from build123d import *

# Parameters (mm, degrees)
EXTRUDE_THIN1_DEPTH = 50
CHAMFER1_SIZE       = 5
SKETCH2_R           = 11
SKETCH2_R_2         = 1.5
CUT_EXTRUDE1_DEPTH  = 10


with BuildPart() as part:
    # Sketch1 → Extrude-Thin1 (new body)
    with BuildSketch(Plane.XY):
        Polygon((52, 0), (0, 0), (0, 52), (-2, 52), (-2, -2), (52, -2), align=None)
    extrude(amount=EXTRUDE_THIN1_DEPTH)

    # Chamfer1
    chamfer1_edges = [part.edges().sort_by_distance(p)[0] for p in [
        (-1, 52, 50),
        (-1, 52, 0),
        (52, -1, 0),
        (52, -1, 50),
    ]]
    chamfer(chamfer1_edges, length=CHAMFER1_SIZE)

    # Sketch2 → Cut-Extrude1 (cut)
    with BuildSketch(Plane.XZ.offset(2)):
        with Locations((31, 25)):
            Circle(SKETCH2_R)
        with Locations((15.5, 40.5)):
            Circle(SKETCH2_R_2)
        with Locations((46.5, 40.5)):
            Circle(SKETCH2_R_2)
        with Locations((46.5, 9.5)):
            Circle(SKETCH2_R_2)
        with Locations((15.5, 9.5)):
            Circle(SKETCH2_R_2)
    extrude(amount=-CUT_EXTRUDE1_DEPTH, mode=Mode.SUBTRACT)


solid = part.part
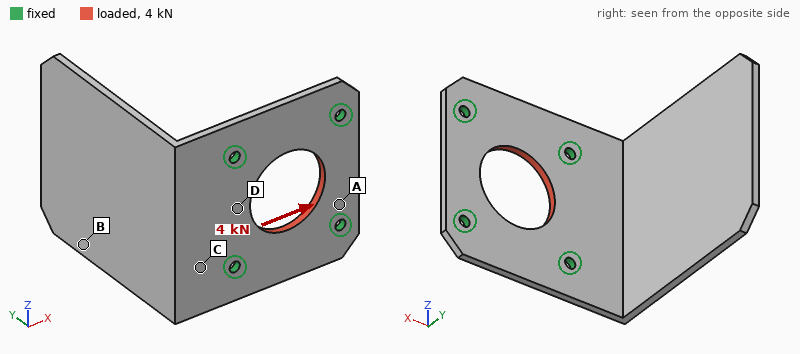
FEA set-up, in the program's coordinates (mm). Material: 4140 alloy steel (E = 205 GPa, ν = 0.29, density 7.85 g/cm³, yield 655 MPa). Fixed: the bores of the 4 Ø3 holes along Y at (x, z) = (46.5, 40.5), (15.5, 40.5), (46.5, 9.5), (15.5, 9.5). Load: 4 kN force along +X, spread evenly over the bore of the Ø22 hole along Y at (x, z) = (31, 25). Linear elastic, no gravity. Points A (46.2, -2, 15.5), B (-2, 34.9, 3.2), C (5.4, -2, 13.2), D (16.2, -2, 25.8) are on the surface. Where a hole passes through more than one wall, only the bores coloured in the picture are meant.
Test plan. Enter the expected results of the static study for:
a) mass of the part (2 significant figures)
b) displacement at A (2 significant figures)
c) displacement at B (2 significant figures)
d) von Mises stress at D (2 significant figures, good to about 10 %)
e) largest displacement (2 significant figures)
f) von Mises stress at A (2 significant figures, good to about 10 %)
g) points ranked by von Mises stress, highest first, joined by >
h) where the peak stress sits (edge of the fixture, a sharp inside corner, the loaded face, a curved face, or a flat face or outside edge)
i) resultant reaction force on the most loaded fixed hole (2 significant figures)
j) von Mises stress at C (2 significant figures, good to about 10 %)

76 g
2.8 µm
1.6 µm
24 MPa
6.3 µm
41 MPa
A > D > C > B
edge of the fixture
1.0 kN
14 MPa
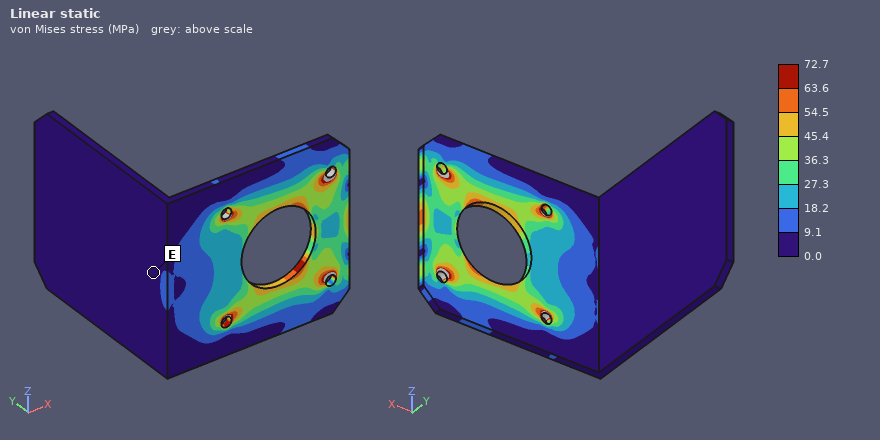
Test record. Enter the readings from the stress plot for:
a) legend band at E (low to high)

0.0 to 9.1 MPa
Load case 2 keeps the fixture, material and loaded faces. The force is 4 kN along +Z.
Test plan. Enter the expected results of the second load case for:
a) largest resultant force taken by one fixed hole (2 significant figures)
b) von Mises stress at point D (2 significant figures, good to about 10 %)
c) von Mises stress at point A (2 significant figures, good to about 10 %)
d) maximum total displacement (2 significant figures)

1.0 kN
33 MPa
37 MPa
4.7 µm
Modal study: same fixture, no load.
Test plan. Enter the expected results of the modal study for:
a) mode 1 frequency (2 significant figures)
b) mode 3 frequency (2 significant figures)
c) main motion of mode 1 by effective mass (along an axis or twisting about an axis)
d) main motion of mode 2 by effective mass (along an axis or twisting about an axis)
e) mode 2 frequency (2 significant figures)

400 Hz
1600 Hz
along X
along Z
1000 Hz
